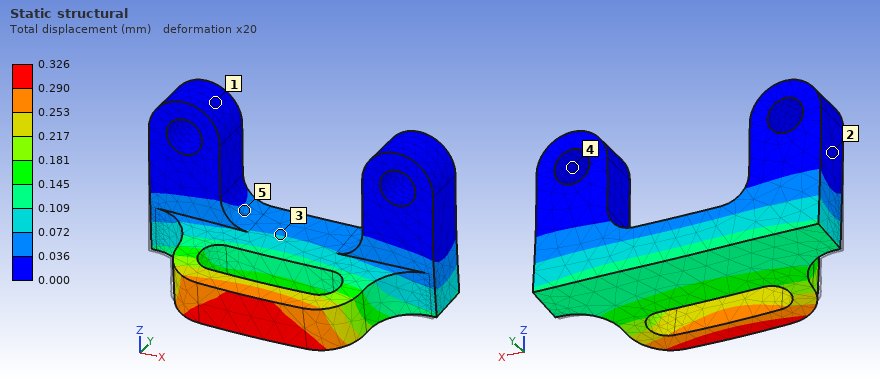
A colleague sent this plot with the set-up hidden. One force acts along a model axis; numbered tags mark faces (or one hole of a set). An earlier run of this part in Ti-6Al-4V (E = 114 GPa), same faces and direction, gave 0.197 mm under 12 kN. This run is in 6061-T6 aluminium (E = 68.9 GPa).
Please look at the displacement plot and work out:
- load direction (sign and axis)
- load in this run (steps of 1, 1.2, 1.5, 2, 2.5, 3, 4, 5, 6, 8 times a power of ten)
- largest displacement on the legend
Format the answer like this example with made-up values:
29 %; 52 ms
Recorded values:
-Z; 12 kN; 0.326 mm
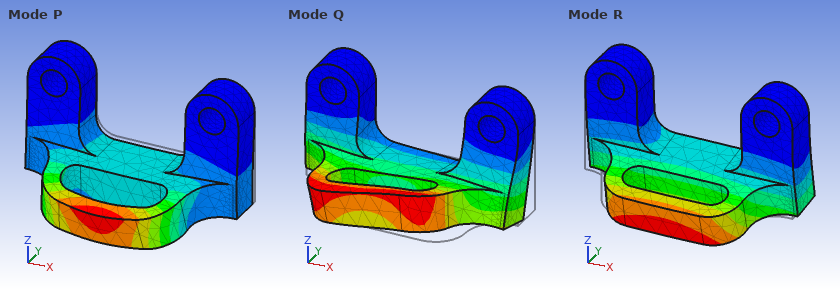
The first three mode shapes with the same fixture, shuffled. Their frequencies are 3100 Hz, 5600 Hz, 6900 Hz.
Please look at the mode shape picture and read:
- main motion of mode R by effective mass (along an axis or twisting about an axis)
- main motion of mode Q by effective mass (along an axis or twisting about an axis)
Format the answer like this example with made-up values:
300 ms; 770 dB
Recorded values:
along Y; along X
